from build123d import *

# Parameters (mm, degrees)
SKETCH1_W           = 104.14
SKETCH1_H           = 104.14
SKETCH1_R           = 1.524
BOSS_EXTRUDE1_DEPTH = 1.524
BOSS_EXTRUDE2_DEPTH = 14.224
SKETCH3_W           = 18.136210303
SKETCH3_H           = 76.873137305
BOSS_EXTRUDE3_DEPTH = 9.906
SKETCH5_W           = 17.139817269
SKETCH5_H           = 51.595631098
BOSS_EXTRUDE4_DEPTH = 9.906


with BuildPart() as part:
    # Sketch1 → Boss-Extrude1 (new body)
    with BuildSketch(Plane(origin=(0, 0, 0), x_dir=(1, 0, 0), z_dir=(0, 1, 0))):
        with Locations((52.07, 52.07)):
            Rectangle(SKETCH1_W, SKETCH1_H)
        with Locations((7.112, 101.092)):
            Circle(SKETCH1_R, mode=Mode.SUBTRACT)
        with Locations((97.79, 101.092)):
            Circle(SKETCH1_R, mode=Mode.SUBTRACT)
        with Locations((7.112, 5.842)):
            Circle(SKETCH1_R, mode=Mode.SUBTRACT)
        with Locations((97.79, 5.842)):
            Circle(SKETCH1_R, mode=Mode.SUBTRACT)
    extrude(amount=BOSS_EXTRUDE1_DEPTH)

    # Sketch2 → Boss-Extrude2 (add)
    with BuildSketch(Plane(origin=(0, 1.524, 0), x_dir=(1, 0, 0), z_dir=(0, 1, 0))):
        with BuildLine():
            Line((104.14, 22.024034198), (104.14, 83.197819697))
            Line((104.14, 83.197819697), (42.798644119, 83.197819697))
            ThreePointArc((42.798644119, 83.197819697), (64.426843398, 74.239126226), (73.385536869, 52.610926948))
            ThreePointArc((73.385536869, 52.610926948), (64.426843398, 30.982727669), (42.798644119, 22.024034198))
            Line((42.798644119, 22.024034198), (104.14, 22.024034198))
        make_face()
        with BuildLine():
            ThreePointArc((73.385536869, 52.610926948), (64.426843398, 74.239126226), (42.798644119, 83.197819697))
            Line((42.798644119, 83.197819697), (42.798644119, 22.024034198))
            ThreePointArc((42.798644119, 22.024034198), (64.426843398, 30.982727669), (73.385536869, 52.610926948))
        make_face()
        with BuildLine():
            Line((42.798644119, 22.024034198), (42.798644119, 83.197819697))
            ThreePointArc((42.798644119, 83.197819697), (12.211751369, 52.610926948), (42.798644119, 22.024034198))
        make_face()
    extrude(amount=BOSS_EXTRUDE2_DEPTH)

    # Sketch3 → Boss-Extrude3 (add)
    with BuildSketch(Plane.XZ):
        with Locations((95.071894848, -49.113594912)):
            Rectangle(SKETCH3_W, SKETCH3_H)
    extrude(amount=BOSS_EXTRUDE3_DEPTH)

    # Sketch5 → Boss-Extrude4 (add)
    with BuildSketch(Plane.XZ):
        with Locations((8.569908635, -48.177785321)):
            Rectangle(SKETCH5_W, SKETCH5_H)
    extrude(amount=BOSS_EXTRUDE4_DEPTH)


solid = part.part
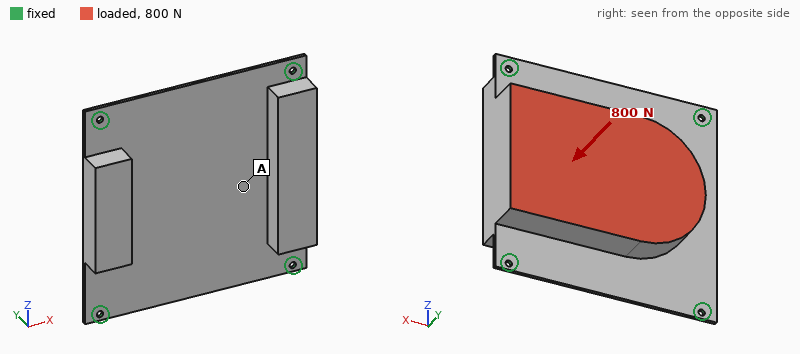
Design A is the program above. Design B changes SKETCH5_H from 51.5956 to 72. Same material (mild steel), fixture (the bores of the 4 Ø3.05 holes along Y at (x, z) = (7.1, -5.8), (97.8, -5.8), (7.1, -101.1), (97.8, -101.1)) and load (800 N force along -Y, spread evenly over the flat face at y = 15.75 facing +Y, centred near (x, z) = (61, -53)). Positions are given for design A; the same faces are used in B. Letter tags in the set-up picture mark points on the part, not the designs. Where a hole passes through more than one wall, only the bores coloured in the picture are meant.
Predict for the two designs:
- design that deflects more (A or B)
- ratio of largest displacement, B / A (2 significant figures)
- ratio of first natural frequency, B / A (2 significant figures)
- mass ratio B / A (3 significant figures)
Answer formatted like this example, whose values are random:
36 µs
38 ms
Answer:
A
0.48
1.4
1.03
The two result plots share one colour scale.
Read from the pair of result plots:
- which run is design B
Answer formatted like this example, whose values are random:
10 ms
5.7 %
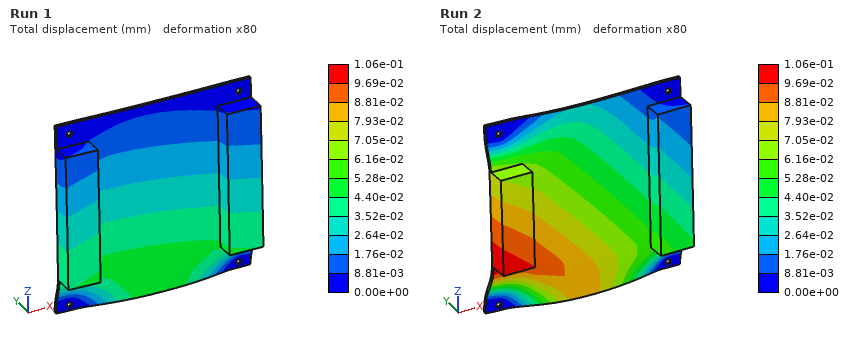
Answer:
Run 1
